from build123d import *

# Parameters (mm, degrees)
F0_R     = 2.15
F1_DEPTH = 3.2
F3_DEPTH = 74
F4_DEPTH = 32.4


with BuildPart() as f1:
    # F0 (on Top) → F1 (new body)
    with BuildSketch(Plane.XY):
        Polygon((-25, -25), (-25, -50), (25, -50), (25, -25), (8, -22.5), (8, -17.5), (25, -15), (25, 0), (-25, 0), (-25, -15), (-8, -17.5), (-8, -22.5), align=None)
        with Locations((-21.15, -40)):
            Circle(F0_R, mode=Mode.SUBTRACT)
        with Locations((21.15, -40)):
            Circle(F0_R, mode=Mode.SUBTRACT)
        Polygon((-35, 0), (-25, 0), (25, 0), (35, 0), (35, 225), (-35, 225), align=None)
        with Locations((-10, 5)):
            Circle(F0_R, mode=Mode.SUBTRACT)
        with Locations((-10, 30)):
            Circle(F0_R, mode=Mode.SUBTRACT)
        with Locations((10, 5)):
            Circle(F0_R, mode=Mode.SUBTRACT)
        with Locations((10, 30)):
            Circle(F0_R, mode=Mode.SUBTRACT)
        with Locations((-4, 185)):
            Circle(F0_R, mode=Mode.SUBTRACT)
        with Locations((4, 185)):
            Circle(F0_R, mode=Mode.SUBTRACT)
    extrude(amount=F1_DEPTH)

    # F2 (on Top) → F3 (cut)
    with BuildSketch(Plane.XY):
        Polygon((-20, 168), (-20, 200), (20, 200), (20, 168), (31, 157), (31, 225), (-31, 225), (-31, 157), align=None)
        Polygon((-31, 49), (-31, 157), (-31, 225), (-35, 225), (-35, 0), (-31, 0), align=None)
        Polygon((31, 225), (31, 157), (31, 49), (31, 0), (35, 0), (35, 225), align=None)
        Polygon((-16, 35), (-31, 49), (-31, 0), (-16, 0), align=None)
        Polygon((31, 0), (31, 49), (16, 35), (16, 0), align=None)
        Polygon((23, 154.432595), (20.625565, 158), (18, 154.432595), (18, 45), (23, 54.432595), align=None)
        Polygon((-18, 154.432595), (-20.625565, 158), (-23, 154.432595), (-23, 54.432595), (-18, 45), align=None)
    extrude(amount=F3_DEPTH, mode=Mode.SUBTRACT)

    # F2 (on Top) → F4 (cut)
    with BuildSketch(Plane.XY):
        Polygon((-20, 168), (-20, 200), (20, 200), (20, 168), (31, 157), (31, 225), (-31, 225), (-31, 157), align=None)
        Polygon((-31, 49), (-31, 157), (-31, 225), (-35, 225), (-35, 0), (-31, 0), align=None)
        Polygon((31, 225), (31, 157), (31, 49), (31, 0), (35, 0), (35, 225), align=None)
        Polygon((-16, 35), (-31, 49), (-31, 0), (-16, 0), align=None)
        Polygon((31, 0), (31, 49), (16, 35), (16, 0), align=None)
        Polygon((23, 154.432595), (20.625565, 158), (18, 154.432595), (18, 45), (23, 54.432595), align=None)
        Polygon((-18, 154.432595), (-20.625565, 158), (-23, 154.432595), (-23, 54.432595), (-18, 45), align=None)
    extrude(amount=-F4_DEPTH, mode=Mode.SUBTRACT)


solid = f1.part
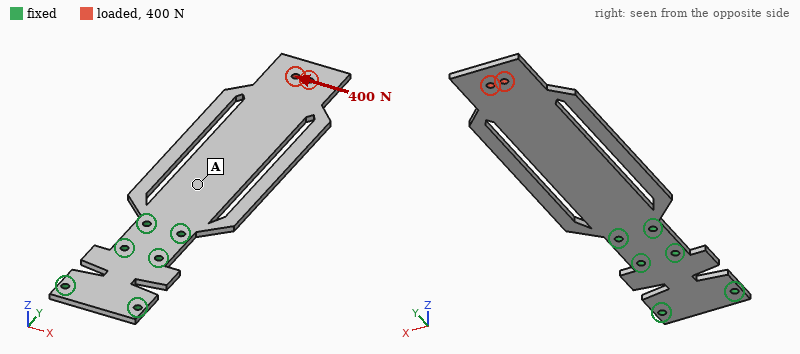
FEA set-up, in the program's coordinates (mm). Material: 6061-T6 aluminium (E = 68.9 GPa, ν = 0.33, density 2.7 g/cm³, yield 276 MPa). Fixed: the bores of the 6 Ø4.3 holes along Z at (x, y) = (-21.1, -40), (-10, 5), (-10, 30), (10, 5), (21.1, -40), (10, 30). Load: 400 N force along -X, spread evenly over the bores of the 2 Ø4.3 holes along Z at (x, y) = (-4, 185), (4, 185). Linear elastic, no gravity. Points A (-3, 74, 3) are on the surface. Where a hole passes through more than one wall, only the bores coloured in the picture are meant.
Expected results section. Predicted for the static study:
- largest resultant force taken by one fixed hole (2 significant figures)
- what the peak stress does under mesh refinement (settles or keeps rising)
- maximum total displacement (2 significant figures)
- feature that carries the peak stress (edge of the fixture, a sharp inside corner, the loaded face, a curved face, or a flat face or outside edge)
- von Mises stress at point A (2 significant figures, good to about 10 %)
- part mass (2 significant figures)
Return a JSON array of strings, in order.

["2.6 kN", "keeps rising", "0.52 mm", "edge of the fixture", "11 MPa", "98 g"]
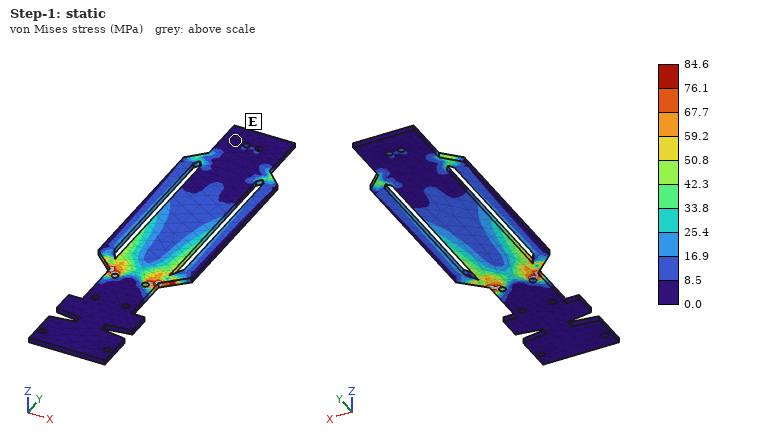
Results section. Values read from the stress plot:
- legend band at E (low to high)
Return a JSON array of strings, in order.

["0.0 to 8.5 MPa"]
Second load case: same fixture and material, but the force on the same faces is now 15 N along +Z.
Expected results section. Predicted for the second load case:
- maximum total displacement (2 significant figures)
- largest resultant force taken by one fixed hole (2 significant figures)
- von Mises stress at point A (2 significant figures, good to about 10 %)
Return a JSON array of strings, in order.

["2.4 mm", "13 N", "19 MPa"]
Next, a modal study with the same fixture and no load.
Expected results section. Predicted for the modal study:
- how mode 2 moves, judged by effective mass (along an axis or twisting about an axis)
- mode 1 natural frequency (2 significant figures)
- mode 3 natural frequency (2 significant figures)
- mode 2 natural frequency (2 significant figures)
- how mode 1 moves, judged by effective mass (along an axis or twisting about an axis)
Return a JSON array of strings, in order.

["twisting about Y", "93 Hz", "570 Hz", "520 Hz", "along Z"]
